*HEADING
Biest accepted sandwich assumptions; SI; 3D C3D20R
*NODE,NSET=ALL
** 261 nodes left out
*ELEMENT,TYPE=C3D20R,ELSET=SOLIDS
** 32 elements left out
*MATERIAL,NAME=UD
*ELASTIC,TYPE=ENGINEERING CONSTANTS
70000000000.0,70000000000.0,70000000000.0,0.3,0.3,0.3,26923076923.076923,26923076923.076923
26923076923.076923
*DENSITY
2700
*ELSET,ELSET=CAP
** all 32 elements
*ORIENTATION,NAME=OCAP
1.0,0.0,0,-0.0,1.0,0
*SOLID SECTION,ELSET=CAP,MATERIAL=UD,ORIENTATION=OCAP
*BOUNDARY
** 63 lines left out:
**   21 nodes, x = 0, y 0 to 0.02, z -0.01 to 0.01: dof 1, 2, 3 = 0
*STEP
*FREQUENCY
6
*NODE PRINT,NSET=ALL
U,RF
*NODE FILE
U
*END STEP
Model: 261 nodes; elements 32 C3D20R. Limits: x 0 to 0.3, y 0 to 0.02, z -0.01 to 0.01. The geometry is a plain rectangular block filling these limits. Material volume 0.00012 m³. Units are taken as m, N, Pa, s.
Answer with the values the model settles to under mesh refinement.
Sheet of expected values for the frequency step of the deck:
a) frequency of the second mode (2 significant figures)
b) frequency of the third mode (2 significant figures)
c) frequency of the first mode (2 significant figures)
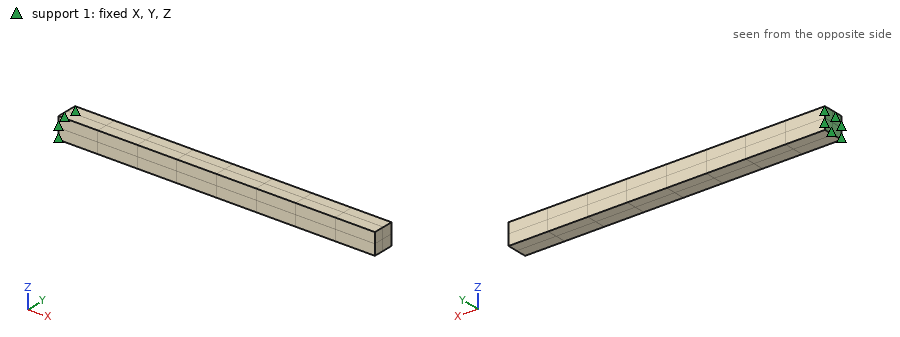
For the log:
180 Hz
1100 Hz
180 Hz
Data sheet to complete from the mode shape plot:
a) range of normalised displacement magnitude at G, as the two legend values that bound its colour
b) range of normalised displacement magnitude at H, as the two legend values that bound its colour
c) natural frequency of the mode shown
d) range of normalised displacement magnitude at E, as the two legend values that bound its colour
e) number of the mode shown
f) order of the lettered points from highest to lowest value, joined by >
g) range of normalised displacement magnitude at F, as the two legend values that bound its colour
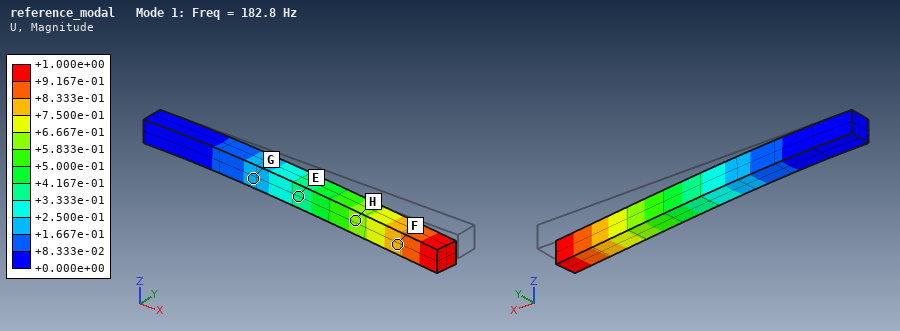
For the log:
+1.667e-01 to +2.500e-01
+5.833e-01 to +6.667e-01
182.8 Hz
+3.333e-01 to +4.167e-01
1
F > H > E > G
+7.500e-01 to +8.333e-01
